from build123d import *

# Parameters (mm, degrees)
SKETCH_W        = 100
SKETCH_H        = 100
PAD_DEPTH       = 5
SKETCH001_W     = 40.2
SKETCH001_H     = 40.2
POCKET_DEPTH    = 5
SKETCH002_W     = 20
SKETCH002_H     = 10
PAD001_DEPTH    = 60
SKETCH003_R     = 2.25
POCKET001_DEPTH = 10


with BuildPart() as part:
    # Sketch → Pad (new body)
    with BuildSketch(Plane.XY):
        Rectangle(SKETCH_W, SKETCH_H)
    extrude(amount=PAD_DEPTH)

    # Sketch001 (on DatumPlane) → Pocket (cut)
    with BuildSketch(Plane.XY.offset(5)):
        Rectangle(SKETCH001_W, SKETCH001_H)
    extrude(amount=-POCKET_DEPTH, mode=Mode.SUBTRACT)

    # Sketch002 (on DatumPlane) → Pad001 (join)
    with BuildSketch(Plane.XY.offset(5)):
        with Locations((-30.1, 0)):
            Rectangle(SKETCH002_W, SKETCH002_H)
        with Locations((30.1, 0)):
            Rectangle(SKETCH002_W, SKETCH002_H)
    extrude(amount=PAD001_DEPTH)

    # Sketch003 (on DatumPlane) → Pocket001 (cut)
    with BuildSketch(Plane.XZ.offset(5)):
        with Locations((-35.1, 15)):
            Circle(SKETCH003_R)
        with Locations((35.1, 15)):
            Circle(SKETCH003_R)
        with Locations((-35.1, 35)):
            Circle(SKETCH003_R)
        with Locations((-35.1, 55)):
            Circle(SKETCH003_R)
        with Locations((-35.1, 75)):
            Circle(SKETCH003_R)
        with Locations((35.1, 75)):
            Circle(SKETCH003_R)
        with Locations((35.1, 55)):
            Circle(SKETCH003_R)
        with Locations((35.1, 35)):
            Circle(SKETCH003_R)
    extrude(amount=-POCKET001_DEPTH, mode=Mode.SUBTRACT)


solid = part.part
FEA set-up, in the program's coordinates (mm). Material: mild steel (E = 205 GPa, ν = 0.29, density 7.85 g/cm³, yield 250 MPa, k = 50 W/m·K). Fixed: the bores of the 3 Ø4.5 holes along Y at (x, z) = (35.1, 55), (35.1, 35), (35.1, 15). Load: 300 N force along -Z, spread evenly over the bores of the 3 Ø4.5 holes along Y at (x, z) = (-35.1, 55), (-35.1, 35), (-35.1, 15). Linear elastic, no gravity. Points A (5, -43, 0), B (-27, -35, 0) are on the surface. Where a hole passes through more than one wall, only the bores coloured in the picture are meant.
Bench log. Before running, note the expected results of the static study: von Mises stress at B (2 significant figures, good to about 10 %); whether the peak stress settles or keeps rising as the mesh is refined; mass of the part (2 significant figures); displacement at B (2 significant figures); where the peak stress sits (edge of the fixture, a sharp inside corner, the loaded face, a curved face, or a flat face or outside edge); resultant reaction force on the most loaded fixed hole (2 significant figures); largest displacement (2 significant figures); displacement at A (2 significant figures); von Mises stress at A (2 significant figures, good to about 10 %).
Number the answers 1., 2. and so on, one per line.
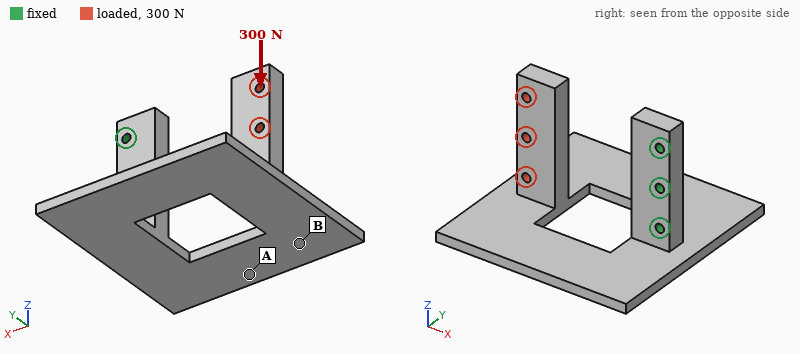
1. 15 MPa
2. keeps rising
3. 510 g
4. 0.31 mm
5. a sharp inside corner
6. 820 N
7. 0.62 mm
8. 0.11 mm
9. 47 MPa
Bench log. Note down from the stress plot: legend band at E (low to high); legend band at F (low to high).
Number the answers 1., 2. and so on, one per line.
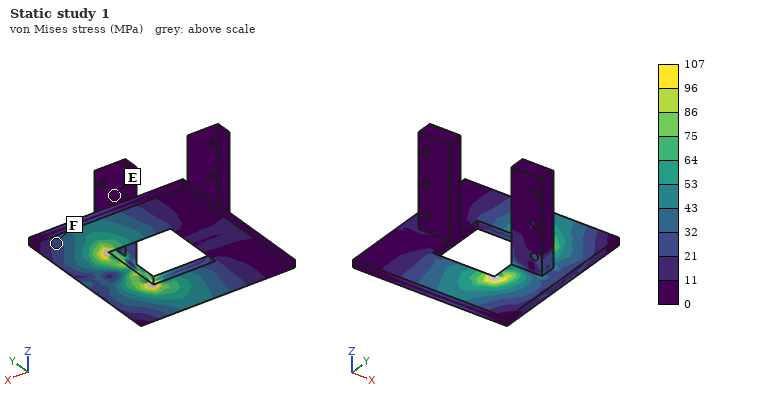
1. 0 to 11 MPa
2. 21 to 32 MPa
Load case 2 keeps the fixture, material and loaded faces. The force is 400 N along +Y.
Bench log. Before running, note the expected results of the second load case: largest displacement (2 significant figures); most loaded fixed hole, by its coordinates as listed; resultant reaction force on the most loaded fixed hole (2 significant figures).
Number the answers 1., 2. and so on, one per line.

1. 0.45 mm
2. (35.1, 15)
3. 270 N
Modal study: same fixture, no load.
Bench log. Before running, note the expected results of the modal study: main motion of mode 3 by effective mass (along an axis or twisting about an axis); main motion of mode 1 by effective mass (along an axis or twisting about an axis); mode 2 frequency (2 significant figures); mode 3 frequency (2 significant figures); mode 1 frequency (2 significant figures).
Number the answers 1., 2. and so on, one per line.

1. along Y
2. along Z
3. 470 Hz
4. 710 Hz
5. 280 Hz
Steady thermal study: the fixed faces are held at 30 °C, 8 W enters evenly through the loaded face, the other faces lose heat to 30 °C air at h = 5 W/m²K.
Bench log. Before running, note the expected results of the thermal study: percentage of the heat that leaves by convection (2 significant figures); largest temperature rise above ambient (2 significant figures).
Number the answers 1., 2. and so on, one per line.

1. 43 %
2. 70 K
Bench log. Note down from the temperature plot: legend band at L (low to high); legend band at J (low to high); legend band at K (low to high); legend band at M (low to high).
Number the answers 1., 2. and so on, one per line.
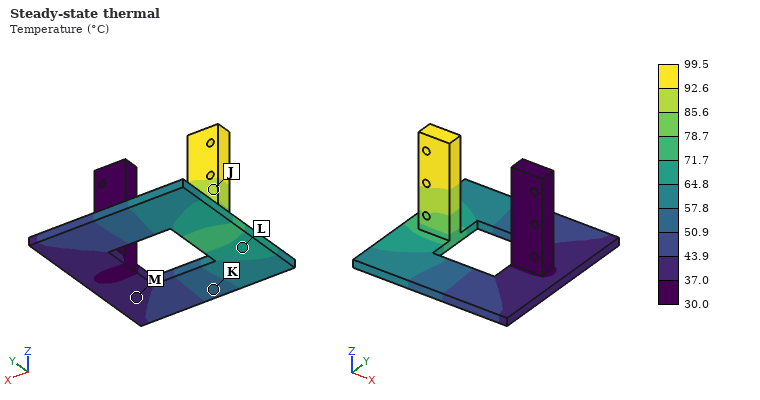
1. 64.8 to 71.7 °C
2. 85.6 to 92.6 °C
3. 50.9 to 57.8 °C
4. 37.0 to 43.9 °C
